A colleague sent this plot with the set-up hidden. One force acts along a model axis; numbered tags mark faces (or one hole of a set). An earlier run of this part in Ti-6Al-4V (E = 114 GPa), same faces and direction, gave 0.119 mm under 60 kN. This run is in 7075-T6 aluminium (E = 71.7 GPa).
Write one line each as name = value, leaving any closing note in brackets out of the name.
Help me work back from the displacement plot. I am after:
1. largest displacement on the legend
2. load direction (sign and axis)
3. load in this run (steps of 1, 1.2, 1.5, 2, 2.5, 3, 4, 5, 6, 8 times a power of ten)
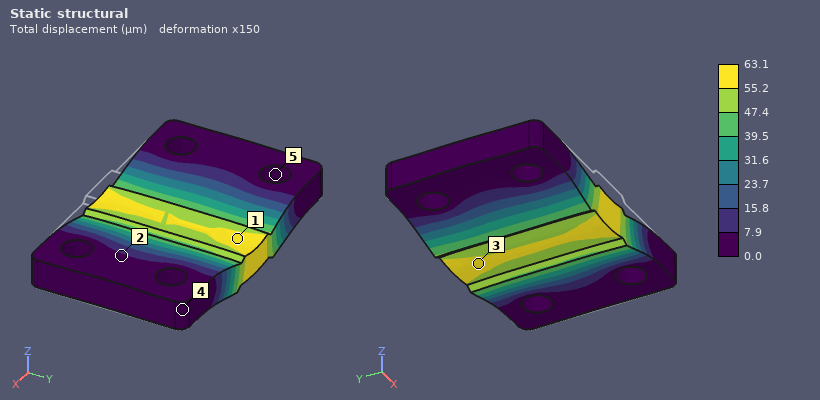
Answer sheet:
largest displacement on the legend = 63.1 µm
load direction = -Z
load in this run = 20 kN
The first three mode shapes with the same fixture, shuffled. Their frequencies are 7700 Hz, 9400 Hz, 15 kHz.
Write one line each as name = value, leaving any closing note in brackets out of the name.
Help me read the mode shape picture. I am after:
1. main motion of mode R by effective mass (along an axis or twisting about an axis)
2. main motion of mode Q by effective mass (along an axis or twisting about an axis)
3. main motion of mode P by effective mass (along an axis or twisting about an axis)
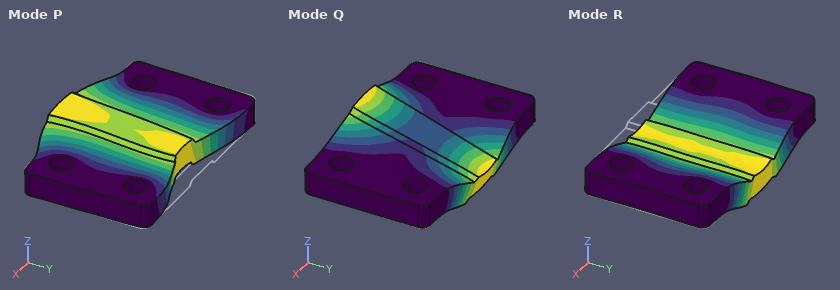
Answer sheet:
main motion of mode R by effective mass = along Z
main motion of mode Q by effective mass = twisting about X
main motion of mode P by effective mass = along Y
